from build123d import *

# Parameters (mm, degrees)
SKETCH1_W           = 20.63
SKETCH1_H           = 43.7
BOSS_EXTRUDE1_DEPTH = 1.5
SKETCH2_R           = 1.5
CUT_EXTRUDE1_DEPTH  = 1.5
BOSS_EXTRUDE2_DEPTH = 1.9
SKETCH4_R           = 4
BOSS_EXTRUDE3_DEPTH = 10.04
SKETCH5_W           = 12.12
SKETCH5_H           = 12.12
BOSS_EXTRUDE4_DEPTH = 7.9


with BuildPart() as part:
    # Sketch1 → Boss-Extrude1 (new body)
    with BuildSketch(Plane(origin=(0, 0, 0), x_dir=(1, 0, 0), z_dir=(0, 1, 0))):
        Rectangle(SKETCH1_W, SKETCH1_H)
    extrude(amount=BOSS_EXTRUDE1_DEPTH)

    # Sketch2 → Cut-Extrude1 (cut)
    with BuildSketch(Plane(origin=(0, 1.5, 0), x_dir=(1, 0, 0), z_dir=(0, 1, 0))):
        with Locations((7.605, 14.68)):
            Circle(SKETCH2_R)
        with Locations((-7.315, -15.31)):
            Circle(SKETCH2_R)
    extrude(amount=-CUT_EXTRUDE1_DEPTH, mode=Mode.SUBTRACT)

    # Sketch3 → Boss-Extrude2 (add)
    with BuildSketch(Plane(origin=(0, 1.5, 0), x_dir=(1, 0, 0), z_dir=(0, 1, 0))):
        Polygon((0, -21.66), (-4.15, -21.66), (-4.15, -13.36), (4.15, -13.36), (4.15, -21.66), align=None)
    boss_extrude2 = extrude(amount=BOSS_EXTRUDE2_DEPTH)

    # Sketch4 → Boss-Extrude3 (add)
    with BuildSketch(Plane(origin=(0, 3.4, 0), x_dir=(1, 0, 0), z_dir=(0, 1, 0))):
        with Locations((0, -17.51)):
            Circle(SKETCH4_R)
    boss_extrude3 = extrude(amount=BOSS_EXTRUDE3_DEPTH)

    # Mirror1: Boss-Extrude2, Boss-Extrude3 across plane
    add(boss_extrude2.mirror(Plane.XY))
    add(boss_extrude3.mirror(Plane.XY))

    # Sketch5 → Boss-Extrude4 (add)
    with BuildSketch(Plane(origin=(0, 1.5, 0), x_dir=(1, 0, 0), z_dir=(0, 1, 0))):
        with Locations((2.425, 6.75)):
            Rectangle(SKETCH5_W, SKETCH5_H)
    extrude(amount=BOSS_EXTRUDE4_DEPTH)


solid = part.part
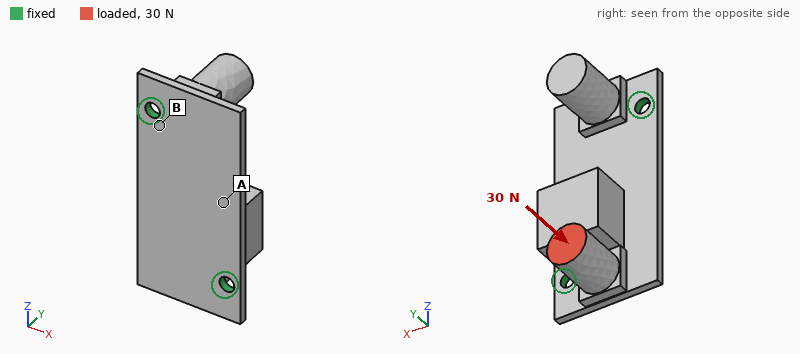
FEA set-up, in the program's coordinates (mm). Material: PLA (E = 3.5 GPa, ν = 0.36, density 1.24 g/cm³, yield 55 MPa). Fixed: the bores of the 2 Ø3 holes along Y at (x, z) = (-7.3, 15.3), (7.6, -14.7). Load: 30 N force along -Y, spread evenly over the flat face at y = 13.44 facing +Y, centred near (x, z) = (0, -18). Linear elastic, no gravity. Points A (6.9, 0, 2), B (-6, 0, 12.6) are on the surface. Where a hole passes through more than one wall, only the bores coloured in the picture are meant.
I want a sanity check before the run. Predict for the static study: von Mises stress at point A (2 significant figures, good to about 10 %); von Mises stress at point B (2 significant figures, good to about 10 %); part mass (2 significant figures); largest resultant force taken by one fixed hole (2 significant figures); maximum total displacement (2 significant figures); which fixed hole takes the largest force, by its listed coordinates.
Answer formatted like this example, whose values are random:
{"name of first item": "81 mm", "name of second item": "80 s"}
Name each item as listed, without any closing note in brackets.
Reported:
{"von Mises stress at point A": "2.0 MPa", "von Mises stress at point B": "4.3 MPa", "part mass": "4.7 g", "largest resultant force taken by one fixed hole": "30 N", "maximum total displacement": "0.37 mm", "which fixed hole takes the largest force, by its listed coordinates": "(7.6, -14.7)"}
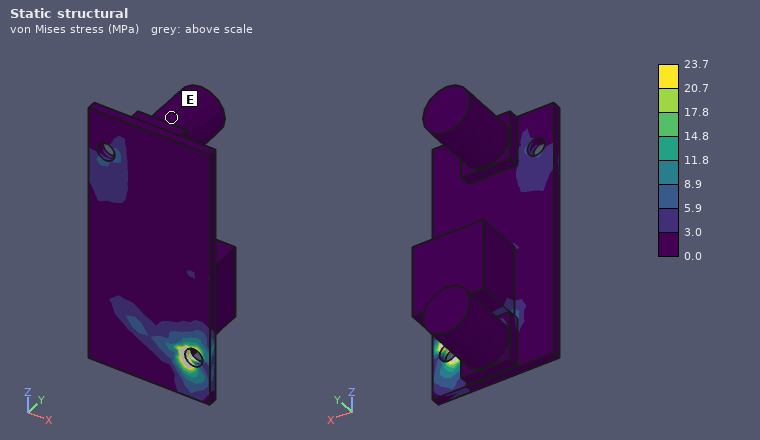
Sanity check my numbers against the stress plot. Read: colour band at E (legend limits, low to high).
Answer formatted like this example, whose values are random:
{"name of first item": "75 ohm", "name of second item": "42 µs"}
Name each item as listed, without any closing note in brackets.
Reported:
{"colour band at E": "0.0 to 3.0 MPa"}
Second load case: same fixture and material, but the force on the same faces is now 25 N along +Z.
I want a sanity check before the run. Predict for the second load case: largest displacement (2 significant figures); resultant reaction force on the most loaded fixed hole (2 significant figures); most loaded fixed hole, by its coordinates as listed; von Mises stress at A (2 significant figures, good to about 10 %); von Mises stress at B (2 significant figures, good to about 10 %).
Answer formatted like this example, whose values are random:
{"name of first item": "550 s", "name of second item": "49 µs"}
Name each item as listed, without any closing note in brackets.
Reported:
{"largest displacement": "0.45 mm", "resultant reaction force on the most loaded fixed hole": "16 N", "most loaded fixed hole, by its coordinates as listed": "(7.6, -14.7)", "von Mises stress at A": "3.6 MPa", "von Mises stress at B": "6.8 MPa"}
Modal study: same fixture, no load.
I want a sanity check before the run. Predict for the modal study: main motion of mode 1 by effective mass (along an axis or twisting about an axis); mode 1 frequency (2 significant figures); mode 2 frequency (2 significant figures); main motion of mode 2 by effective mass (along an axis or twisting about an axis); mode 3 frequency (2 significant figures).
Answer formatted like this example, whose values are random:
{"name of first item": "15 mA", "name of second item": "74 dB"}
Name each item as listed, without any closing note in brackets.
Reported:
{"main motion of mode 1 by effective mass": "along X", "mode 1 frequency": "1100 Hz", "mode 2 frequency": "1300 Hz", "main motion of mode 2 by effective mass": "along Y", "mode 3 frequency": "1600 Hz"}
